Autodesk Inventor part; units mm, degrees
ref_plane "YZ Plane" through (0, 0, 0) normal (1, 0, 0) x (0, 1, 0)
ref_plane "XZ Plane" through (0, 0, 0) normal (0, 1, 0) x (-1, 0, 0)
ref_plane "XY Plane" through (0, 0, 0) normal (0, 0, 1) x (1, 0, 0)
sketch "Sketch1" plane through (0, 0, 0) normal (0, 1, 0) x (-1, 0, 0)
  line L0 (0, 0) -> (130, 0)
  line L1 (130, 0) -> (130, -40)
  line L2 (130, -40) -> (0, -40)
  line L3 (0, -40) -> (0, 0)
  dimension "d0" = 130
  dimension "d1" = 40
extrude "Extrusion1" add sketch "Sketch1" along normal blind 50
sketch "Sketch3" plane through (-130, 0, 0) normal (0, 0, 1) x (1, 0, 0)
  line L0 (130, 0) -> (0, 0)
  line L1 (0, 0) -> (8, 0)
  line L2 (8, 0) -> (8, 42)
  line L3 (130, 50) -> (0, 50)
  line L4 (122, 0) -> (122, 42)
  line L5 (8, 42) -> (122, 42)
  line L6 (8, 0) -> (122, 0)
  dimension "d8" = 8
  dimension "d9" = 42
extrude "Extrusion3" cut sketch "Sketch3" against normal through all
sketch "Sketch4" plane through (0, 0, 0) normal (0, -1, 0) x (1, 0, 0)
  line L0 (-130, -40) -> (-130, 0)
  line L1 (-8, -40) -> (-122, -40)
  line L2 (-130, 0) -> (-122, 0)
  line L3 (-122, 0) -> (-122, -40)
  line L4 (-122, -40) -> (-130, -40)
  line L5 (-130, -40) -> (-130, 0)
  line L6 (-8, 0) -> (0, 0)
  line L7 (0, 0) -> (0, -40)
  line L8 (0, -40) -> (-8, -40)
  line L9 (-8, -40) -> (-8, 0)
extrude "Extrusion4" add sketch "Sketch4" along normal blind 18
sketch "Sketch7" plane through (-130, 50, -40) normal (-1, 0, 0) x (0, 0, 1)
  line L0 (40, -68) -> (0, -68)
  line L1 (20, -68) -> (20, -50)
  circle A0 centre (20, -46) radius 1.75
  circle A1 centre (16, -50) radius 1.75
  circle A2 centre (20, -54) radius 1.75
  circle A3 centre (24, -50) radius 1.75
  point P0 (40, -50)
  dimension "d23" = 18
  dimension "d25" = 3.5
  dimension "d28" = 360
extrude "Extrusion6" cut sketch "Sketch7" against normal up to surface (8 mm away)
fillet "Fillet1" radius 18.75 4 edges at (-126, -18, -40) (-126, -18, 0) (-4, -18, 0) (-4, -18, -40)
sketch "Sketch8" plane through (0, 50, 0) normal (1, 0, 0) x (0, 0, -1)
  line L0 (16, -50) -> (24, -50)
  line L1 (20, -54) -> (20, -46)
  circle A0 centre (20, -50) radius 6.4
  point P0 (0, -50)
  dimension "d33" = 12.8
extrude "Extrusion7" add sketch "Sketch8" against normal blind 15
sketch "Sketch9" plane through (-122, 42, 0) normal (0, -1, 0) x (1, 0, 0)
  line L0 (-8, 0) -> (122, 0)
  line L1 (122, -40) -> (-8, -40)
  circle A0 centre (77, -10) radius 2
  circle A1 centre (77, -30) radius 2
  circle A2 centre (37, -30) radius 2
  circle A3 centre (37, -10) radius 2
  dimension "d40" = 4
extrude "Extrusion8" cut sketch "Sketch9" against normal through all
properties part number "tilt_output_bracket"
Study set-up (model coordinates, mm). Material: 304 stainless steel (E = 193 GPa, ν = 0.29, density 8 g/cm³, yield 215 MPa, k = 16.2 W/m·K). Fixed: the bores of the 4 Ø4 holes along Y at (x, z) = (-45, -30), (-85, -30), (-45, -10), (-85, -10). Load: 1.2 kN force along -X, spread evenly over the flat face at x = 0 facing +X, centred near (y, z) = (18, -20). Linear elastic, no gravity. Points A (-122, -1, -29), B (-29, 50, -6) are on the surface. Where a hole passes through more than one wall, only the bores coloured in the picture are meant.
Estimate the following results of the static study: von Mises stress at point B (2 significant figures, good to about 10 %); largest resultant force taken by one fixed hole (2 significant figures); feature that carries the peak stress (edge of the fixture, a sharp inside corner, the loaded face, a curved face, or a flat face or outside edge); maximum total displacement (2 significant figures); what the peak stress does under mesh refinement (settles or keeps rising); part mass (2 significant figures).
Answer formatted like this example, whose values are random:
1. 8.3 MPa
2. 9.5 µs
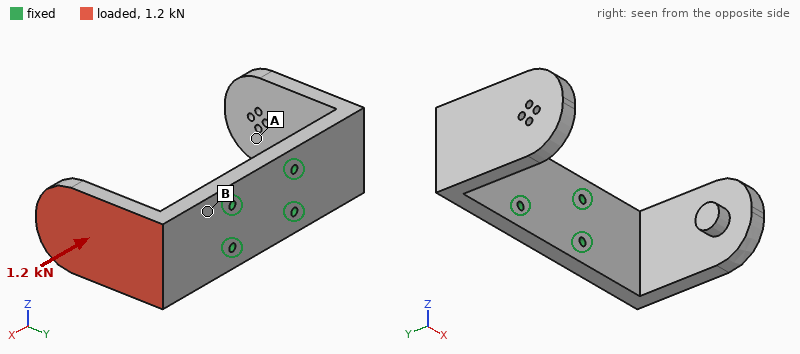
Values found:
1. 74 MPa
2. 560 N
3. edge of the fixture
4. 0.37 mm
5. keeps rising
6. 620 g
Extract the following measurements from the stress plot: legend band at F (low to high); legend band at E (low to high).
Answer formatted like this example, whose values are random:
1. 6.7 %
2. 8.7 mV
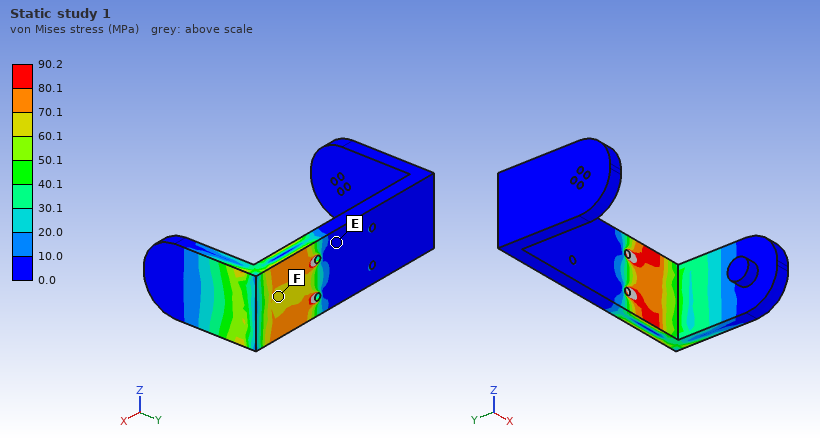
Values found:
1. 60.1 to 70.1 MPa
2. 0.0 to 10.0 MPa
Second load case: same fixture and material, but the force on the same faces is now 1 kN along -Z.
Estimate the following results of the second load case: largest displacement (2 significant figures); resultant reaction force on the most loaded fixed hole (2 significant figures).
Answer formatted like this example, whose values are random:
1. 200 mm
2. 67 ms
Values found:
1. 0.12 mm
2. 2.0 kN
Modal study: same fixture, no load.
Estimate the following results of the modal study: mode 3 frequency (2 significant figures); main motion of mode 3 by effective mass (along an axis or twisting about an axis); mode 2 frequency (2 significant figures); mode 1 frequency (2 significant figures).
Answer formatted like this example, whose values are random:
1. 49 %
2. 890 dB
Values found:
1. 1300 Hz
2. along Z
3. 820 Hz
4. 780 Hz
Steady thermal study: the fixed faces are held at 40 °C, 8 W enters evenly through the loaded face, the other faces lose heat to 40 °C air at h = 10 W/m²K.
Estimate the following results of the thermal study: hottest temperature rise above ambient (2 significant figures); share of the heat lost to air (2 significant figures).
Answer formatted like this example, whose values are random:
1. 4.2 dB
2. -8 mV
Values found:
1. 67 K
2. 39 %
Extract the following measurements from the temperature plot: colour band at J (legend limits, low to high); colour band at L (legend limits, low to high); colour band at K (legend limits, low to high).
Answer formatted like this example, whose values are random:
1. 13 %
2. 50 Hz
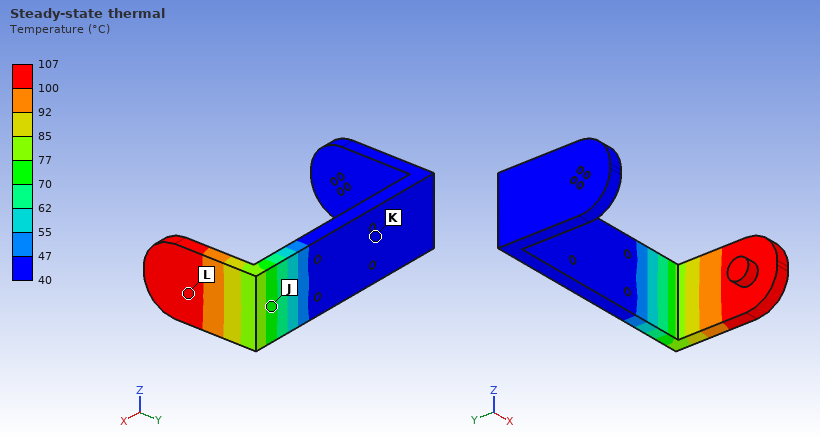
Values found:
1. 70 to 77 °C
2. 100 to 107 °C
3. 40 to 47 °C
